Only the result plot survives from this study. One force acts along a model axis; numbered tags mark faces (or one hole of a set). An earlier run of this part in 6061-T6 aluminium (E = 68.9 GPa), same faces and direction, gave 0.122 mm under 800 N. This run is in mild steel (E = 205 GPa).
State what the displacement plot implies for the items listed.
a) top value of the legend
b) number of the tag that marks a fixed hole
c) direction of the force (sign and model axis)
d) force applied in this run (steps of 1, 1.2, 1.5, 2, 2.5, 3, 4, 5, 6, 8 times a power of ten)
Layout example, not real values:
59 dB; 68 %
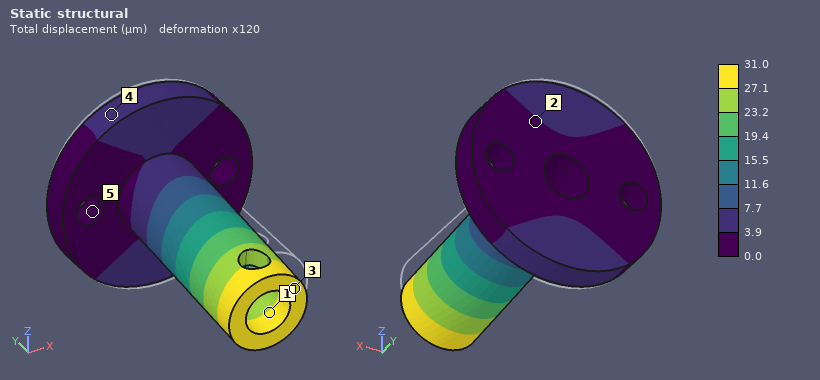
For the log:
31.0 µm; 5; -Z; 600 N
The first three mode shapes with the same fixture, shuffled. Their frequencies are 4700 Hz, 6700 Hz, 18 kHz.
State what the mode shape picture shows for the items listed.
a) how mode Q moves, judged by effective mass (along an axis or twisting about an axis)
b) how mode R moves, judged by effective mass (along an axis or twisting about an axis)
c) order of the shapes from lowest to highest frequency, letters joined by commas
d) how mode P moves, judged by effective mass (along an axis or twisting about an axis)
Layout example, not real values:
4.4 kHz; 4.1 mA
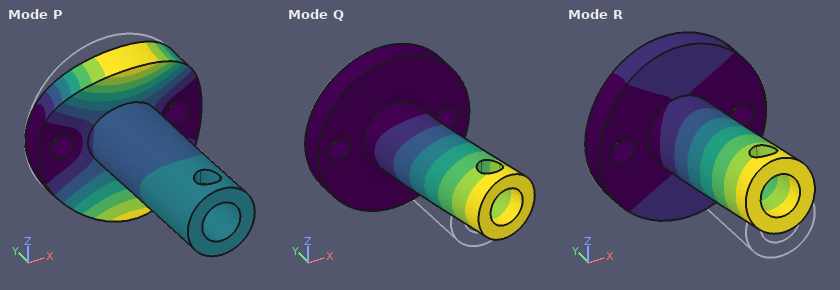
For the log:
along X; along Z; R, Q, P; along Y
